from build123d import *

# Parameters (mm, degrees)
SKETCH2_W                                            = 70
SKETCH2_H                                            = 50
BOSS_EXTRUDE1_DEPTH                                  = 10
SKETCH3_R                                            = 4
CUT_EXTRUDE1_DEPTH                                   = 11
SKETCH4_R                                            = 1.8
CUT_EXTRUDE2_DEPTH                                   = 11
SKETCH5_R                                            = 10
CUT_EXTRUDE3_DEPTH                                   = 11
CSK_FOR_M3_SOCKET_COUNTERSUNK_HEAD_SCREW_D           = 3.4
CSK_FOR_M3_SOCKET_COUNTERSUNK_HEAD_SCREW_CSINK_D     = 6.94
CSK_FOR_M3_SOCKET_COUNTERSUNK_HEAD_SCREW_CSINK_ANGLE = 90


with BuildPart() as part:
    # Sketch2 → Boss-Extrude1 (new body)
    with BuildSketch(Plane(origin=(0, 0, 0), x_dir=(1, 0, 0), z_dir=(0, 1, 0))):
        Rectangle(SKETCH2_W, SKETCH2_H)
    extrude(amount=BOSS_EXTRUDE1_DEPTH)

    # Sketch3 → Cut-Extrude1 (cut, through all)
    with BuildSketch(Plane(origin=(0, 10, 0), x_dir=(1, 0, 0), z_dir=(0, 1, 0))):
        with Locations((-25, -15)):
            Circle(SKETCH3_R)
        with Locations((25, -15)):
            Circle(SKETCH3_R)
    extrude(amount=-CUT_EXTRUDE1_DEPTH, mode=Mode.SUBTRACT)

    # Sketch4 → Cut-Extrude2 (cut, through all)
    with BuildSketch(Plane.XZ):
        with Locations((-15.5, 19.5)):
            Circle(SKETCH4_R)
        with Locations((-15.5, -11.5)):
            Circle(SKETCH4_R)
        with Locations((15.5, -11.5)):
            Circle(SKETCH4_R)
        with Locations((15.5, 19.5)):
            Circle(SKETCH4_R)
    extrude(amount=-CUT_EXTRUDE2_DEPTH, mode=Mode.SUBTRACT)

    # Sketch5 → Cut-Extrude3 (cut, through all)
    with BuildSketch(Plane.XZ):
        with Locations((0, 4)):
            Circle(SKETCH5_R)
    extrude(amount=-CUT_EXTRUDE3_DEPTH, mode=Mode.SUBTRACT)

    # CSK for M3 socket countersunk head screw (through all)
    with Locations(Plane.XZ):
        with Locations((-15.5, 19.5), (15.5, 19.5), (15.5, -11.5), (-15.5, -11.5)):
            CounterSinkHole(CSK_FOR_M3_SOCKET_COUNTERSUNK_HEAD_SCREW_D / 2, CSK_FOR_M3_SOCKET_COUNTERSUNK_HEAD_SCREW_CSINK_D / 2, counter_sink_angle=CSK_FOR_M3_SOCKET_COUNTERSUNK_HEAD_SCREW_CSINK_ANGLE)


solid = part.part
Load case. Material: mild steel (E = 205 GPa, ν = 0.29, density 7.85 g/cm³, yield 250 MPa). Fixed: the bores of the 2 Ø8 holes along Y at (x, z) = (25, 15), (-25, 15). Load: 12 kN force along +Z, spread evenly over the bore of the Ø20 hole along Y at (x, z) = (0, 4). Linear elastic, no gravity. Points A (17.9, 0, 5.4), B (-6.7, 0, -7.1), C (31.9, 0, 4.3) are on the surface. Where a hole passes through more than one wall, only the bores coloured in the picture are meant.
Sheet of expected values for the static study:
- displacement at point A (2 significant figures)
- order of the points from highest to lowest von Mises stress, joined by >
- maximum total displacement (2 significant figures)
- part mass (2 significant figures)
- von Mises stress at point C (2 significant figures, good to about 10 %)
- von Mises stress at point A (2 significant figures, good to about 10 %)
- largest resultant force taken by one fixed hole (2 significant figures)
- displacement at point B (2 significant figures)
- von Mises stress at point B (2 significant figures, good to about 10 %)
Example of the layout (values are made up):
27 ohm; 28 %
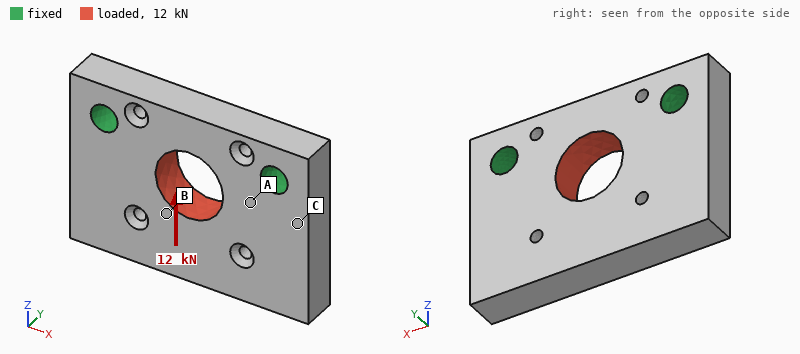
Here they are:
2.3 µm; A > B > C; 6.7 µm; 240 g; 11 MPa; 37 MPa; 6.1 kN; 4.5 µm; 24 MPa
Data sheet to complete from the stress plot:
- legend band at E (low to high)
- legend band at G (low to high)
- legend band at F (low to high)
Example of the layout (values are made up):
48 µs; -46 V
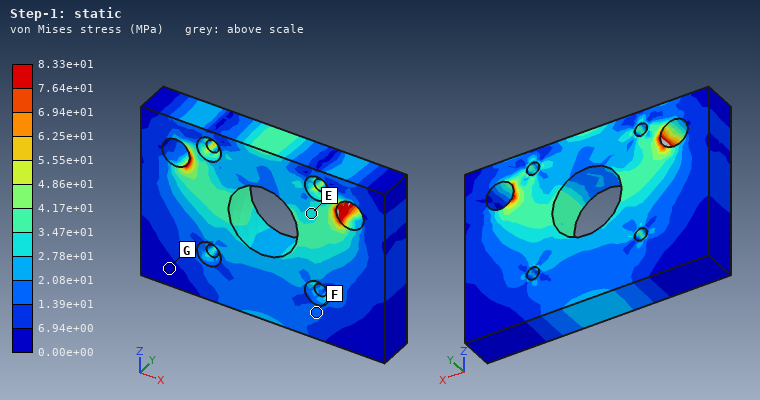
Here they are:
2.78e+01 to 3.47e+01 MPa; 0.00e+00 to 6.94e+00 MPa; 1.39e+01 to 2.08e+01 MPa
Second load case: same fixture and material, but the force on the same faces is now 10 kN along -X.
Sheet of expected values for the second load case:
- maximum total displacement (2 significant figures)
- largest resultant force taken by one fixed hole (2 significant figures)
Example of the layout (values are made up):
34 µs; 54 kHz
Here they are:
5.9 µm; 5.2 kN
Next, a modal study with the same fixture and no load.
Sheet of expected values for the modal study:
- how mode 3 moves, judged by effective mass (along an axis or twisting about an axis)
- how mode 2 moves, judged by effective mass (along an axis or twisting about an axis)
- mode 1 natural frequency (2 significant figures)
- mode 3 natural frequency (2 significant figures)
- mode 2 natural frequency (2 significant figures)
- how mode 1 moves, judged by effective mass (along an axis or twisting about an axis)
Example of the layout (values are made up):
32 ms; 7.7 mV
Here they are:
along X; twisting about Z; 4400 Hz; 13 kHz; 7800 Hz; along Y
